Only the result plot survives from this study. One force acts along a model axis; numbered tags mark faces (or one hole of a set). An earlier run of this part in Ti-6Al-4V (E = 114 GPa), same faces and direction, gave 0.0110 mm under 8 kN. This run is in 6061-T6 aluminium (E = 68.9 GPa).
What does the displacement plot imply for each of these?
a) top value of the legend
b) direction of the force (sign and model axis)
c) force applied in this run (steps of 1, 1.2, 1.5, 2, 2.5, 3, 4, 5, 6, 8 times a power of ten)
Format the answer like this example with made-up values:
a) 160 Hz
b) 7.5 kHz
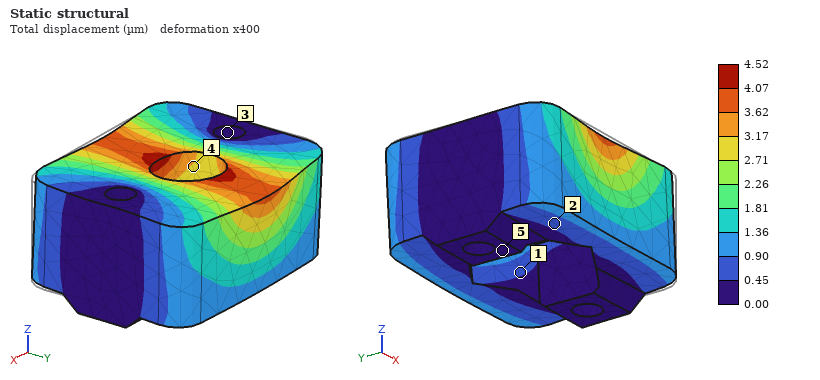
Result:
a) 4.52 µm
b) +Y
c) 2 kN
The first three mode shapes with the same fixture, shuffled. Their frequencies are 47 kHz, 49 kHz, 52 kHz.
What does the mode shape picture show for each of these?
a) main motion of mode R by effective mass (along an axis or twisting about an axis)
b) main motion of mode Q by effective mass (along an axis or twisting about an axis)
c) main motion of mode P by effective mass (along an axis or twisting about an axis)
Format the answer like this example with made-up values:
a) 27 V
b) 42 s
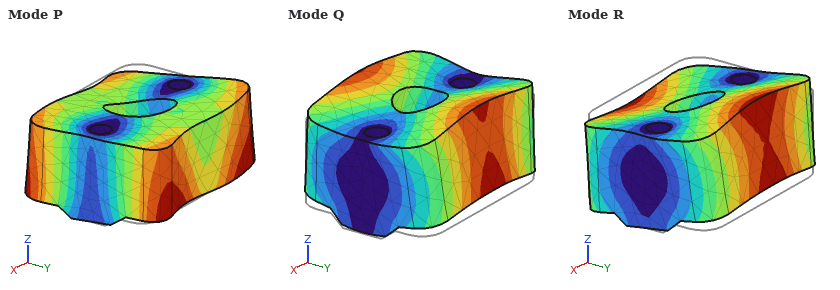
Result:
a) twisting about X
b) along Z
c) twisting about Z
